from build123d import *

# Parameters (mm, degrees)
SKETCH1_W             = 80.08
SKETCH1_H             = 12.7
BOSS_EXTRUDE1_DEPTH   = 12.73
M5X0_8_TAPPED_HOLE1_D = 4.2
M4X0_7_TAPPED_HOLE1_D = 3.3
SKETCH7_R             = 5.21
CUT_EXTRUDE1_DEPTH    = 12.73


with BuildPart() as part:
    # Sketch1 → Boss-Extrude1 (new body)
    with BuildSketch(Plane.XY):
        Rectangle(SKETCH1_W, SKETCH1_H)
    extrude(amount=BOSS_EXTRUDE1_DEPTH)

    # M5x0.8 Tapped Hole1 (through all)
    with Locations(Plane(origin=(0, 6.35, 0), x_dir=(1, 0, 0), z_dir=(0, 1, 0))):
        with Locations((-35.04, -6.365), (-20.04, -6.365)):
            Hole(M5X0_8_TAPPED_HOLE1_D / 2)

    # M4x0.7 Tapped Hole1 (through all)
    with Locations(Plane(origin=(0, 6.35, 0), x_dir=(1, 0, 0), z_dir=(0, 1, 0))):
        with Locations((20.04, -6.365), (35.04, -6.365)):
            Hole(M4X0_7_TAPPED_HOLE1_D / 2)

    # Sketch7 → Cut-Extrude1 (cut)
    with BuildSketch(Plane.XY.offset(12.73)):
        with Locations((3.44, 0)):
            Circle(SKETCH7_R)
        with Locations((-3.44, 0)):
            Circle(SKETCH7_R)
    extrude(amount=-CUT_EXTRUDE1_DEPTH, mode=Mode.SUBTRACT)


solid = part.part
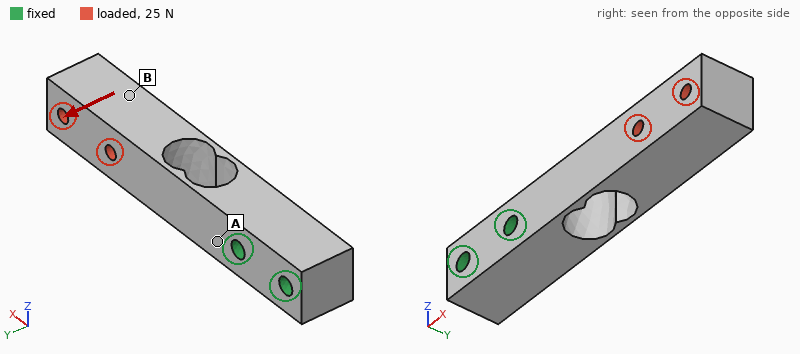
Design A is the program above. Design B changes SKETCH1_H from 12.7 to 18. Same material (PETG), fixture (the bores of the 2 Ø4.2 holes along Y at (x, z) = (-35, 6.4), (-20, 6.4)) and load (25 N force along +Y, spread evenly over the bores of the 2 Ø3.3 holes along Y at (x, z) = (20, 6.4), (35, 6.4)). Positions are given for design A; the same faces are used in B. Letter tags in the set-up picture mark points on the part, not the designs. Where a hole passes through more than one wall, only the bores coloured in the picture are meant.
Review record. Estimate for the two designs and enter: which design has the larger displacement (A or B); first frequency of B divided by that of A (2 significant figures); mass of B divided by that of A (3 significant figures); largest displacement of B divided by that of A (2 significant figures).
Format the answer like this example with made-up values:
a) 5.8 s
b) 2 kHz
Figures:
a) A
b) 1.5
c) 1.49
d) 0.18
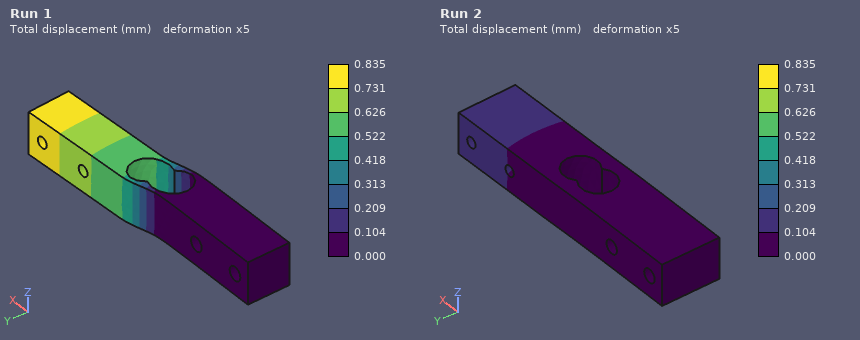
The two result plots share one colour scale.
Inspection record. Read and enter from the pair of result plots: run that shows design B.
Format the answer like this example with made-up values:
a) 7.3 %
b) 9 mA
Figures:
a) Run 2
